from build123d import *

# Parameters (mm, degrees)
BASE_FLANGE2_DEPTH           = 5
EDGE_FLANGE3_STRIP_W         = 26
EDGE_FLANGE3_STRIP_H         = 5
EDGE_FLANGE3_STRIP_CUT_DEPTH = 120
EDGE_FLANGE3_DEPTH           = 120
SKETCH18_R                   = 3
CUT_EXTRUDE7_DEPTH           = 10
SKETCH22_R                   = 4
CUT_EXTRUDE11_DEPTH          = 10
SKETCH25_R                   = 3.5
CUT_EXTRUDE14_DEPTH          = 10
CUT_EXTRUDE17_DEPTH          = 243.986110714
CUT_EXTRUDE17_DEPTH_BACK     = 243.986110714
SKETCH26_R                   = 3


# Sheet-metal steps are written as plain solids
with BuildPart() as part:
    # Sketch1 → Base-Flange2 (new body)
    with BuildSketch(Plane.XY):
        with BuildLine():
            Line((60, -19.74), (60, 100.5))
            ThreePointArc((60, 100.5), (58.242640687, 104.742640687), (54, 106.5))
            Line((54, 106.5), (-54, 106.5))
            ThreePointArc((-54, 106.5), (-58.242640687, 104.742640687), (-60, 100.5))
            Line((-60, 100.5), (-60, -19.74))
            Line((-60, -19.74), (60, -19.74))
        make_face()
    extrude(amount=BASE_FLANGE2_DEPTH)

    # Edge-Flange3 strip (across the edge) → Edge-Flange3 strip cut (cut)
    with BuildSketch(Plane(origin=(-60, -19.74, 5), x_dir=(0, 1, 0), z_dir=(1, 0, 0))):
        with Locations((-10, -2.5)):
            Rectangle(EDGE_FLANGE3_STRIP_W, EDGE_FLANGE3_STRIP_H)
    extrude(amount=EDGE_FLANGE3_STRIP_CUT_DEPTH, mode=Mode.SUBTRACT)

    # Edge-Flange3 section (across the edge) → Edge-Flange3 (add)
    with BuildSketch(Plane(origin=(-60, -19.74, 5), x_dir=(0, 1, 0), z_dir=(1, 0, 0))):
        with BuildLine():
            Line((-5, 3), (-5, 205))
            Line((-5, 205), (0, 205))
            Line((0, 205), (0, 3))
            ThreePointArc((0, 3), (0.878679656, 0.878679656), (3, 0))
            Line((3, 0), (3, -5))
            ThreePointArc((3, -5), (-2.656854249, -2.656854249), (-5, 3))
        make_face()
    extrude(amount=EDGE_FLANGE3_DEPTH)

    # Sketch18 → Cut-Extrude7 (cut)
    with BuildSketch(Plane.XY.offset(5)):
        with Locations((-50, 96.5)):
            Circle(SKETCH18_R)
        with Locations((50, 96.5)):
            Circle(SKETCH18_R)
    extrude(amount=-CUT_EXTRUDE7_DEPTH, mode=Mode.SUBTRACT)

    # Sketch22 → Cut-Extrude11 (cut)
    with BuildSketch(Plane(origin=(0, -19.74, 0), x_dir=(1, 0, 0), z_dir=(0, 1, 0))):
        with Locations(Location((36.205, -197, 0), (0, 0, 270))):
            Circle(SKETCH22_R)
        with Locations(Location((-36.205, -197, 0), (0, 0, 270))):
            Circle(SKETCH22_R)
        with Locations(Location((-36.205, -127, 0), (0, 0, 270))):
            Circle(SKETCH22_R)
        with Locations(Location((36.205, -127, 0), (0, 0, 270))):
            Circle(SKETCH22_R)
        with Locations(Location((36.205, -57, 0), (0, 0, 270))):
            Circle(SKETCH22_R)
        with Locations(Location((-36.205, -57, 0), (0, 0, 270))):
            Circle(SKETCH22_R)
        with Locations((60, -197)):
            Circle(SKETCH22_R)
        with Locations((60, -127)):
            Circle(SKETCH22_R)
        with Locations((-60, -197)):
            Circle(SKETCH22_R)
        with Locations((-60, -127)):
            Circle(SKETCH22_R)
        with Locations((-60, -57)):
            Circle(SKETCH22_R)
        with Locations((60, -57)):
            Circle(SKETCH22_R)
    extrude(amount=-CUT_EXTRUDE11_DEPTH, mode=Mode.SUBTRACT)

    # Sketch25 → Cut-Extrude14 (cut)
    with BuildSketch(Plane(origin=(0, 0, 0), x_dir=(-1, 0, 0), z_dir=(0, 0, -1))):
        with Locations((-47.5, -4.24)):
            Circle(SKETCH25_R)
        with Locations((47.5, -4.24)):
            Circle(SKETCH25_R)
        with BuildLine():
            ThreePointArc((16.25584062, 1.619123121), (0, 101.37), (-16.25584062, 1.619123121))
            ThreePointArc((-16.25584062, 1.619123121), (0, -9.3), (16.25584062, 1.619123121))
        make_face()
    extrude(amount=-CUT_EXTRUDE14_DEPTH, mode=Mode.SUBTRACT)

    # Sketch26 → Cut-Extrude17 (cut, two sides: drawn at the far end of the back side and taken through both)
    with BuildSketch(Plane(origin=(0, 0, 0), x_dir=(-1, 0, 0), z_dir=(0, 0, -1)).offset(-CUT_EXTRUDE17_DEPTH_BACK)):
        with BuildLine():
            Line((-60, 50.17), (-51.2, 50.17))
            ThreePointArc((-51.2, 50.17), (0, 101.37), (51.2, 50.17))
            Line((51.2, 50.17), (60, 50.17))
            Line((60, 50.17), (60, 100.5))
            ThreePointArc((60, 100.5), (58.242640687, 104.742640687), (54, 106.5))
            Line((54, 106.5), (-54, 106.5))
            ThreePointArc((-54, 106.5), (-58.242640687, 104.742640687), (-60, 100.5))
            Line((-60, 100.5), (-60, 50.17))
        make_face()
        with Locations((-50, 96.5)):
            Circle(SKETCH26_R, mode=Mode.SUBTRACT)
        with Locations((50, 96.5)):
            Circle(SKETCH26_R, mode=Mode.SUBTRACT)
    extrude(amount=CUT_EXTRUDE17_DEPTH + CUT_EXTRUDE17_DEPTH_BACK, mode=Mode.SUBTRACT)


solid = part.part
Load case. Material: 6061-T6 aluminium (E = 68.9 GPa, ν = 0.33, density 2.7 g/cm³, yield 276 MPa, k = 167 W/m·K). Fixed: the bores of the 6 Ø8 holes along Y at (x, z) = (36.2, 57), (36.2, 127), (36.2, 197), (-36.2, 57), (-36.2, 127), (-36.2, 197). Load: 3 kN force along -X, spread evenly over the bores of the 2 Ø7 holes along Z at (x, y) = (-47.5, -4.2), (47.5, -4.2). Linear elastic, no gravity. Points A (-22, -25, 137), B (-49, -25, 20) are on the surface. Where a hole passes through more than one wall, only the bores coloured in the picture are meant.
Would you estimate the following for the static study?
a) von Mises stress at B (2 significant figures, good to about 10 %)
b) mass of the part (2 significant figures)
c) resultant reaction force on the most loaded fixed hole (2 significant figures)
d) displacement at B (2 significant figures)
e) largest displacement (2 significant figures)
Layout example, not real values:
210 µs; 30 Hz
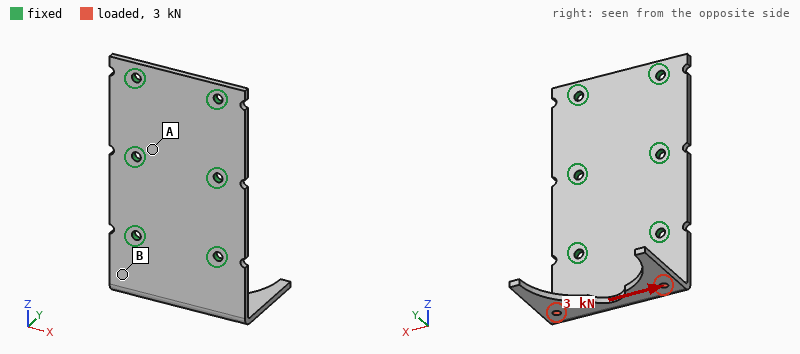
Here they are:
41 MPa; 380 g; 2.4 kN; 0.30 mm; 1.1 mm
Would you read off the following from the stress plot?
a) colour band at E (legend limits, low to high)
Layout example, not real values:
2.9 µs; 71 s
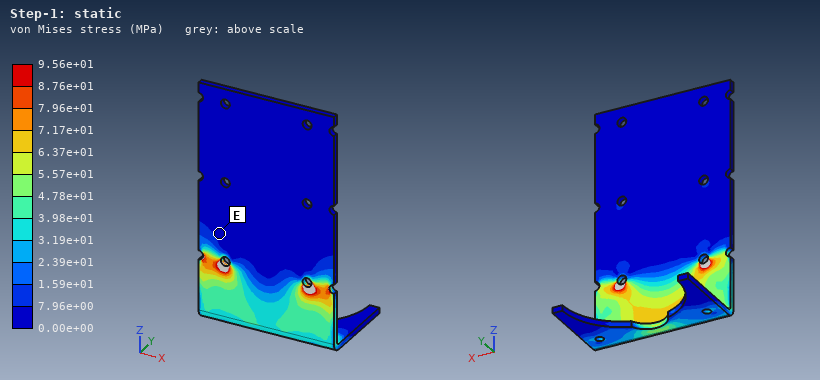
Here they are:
0.00e+00 to 7.96e+00 MPa
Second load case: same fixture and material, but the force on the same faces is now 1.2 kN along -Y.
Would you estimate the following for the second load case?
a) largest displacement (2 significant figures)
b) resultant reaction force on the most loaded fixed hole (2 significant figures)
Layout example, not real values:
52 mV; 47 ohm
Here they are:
1.7 mm; 700 N
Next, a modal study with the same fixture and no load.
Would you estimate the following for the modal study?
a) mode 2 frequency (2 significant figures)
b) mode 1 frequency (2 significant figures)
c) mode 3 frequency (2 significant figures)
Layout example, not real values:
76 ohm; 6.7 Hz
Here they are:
750 Hz; 560 Hz; 1300 Hz
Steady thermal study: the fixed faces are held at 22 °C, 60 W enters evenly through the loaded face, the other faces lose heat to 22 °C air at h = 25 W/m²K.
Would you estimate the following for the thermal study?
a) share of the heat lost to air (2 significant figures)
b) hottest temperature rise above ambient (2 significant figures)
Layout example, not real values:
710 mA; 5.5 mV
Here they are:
26 %; 50 K
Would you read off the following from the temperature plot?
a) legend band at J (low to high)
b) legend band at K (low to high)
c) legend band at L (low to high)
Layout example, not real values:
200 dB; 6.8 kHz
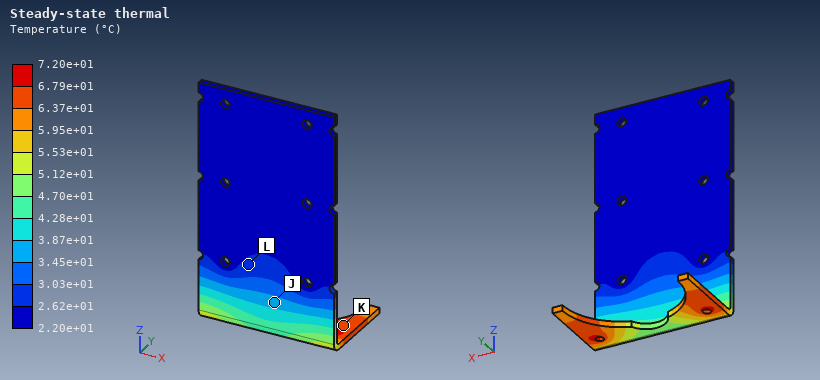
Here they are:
3.45e+01 to 3.87e+01 °C; 6.37e+01 to 6.79e+01 °C; 2.62e+01 to 3.03e+01 °C
